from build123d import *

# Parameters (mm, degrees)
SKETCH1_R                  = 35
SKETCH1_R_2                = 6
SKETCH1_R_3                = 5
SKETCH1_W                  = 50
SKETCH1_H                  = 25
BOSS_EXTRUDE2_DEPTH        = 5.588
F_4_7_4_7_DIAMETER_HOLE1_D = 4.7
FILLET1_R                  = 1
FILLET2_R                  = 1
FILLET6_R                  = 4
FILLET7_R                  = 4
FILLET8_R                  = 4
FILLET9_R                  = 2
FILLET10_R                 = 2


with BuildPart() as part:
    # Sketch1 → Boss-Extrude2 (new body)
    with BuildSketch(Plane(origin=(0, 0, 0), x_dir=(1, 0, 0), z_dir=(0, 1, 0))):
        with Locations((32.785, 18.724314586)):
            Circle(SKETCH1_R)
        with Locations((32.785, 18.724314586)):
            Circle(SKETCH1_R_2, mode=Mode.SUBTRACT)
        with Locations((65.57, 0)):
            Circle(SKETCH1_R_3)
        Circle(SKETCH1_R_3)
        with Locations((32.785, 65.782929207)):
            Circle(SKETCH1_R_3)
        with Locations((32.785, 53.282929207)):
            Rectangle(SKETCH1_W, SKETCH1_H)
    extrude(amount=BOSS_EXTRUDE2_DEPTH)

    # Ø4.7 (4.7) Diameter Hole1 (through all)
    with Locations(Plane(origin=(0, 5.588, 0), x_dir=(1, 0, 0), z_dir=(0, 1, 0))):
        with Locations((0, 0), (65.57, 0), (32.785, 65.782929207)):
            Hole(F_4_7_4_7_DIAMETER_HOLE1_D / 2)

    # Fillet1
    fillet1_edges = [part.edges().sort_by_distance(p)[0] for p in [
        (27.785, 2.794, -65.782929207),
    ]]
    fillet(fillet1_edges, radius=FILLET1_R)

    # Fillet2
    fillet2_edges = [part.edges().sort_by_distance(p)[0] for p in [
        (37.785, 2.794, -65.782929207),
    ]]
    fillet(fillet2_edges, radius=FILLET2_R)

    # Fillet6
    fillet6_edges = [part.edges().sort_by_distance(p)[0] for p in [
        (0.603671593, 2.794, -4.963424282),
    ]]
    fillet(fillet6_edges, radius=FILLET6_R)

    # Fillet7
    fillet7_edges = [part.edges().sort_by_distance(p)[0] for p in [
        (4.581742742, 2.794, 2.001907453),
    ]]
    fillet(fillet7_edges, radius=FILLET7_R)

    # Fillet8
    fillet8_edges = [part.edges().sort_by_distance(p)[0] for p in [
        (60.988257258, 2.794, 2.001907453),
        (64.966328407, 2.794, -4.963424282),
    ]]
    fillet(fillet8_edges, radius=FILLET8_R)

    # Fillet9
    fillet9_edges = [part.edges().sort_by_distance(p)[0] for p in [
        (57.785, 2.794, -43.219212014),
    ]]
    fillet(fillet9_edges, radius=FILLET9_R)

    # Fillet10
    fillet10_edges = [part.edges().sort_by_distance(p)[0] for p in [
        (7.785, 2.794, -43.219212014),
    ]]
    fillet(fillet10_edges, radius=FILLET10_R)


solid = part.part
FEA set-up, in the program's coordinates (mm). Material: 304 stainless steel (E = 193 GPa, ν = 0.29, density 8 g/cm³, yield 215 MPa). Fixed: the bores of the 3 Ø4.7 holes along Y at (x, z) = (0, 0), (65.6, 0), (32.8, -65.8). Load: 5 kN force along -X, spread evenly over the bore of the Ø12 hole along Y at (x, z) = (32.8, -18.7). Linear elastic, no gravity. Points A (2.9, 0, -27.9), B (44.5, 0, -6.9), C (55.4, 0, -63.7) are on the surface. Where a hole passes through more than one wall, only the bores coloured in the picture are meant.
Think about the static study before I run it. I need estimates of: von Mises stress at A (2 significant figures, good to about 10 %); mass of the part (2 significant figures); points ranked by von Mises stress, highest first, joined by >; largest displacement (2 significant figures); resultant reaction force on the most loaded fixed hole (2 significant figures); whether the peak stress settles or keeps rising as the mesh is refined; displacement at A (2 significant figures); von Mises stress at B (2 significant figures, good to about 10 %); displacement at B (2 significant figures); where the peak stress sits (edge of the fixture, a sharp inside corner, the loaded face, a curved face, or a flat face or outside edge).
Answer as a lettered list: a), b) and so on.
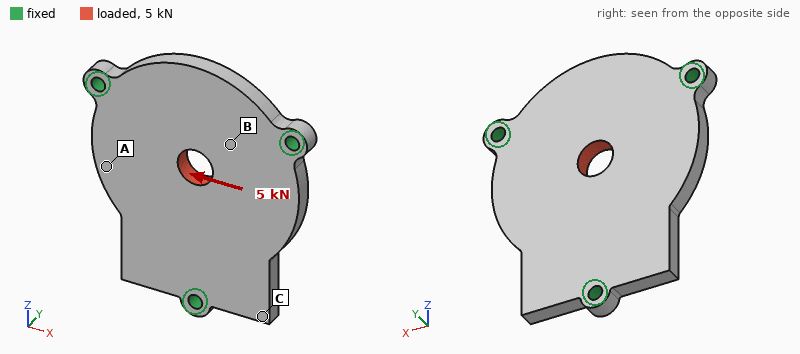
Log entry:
a) 9.6 MPa
b) 210 g
c) B > A > C
d) 5.6 µm
e) 2.1 kN
f) keeps rising
g) 3.9 µm
h) 20 MPa
i) 2.7 µm
j) edge of the fixture
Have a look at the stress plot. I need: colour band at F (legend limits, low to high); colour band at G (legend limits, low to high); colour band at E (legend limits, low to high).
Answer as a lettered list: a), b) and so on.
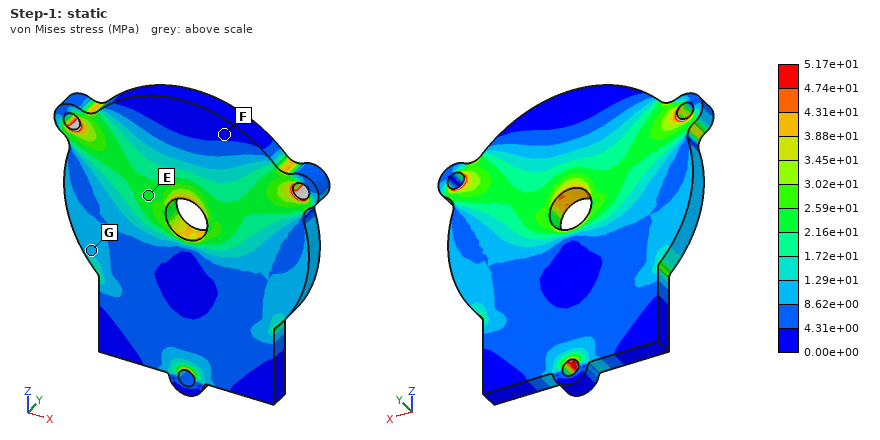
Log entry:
a) 0.00e+00 to 4.31e+00 MPa
b) 8.62e+00 to 1.29e+01 MPa
c) 2.16e+01 to 2.59e+01 MPa
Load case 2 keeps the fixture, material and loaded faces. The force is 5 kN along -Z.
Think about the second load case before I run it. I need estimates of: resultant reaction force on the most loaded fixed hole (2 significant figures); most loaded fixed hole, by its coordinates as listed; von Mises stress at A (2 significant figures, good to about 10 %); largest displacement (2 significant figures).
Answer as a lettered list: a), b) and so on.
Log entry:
a) 2.1 kN
b) (32.8, -65.8)
c) 6.1 MPa
d) 5.5 µm
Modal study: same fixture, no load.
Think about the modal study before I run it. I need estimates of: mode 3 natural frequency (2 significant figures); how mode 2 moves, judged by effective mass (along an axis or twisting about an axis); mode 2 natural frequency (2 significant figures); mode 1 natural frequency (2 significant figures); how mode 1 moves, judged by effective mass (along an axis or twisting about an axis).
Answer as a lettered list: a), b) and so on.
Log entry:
a) 5300 Hz
b) twisting about Z
c) 4700 Hz
d) 4200 Hz
e) along Y
